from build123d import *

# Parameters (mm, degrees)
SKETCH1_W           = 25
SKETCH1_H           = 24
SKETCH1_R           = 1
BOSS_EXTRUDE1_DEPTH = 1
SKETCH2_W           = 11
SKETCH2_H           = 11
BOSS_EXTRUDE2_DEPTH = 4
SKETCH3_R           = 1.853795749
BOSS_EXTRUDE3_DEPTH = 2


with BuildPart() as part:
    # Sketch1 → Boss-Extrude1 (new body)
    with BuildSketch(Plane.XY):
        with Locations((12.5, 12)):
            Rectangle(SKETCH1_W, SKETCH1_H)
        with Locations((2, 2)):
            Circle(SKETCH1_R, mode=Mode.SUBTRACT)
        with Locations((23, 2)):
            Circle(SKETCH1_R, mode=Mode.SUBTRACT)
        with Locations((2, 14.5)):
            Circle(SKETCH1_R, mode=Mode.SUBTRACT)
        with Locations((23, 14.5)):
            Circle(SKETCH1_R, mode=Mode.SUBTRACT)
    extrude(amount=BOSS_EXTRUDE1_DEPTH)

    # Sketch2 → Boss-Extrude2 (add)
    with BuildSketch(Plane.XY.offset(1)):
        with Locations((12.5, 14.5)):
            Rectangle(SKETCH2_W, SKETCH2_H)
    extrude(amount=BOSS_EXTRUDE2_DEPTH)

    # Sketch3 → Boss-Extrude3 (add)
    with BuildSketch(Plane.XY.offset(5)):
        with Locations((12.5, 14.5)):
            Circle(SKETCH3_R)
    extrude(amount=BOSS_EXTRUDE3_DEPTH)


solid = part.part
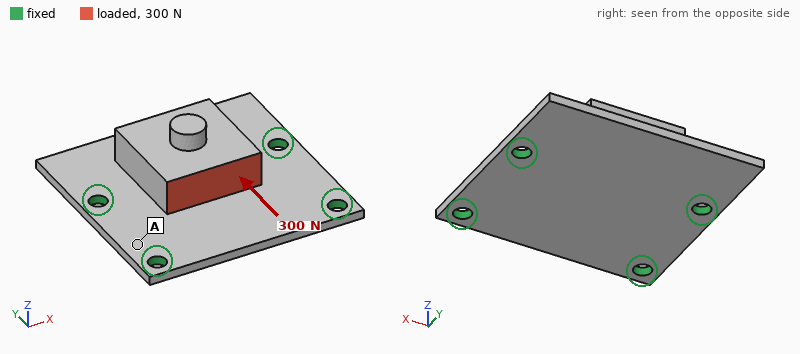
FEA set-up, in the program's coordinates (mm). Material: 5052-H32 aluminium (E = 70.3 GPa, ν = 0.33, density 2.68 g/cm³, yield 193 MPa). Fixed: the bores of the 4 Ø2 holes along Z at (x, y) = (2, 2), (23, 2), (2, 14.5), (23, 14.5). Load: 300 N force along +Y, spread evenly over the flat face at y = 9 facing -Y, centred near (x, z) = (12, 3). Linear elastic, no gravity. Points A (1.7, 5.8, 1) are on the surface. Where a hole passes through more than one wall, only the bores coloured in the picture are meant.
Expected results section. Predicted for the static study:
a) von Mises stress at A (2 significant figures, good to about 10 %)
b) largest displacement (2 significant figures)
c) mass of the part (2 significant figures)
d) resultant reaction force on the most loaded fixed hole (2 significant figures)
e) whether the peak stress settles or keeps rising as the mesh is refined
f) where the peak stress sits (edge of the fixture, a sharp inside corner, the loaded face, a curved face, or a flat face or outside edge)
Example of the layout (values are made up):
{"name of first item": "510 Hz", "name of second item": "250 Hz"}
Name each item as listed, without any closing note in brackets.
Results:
{"von Mises stress at A": "18 MPa", "largest displacement": "50 µm", "mass of the part": "2.9 g", "resultant reaction force on the most loaded fixed hole": "97 N", "whether the peak stress settles or keeps rising as the mesh is refined": "keeps rising", "where the peak stress sits": "edge of the fixture"}
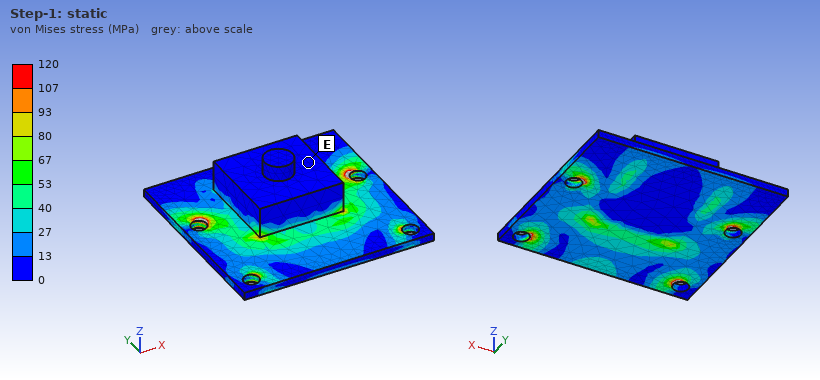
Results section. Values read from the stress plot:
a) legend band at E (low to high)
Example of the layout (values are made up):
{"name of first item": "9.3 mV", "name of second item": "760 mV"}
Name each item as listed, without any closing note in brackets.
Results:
{"legend band at E": "0 to 13 MPa"}
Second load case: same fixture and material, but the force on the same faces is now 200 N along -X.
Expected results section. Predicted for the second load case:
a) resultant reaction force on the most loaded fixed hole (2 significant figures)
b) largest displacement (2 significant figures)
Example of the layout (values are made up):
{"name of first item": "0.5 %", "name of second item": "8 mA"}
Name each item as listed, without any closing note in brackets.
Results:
{"resultant reaction force on the most loaded fixed hole": "77 N", "largest displacement": "6.9 µm"}
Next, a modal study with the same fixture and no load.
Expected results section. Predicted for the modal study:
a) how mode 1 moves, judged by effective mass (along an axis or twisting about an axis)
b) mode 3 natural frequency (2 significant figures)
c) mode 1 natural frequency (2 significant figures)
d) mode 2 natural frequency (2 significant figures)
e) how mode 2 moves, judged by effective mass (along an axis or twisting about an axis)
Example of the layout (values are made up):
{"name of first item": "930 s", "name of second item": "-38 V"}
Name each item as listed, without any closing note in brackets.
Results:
{"how mode 1 moves, judged by effective mass": "along Z", "mode 3 natural frequency": "17 kHz", "mode 1 natural frequency": "8100 Hz", "mode 2 natural frequency": "12 kHz", "how mode 2 moves, judged by effective mass": "along Z"}
